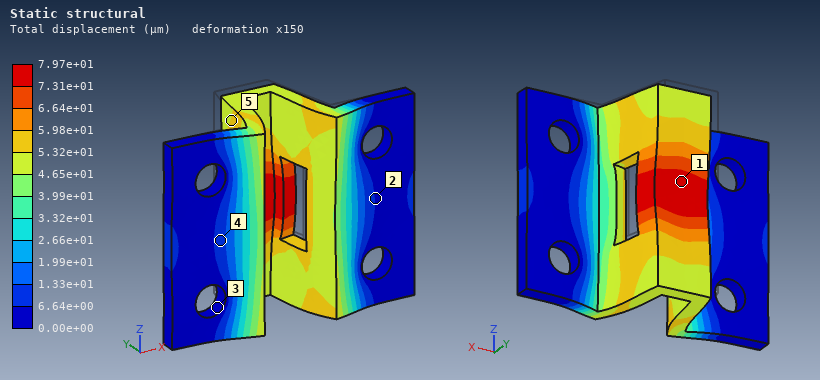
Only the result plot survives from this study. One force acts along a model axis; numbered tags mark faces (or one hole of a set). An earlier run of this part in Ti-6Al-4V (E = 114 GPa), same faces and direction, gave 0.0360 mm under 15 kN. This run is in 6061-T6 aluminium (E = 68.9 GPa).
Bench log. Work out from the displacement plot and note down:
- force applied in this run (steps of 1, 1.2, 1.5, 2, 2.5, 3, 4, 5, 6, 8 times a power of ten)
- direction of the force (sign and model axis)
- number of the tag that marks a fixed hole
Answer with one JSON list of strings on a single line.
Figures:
["20 kN", "-Y", "3"]
